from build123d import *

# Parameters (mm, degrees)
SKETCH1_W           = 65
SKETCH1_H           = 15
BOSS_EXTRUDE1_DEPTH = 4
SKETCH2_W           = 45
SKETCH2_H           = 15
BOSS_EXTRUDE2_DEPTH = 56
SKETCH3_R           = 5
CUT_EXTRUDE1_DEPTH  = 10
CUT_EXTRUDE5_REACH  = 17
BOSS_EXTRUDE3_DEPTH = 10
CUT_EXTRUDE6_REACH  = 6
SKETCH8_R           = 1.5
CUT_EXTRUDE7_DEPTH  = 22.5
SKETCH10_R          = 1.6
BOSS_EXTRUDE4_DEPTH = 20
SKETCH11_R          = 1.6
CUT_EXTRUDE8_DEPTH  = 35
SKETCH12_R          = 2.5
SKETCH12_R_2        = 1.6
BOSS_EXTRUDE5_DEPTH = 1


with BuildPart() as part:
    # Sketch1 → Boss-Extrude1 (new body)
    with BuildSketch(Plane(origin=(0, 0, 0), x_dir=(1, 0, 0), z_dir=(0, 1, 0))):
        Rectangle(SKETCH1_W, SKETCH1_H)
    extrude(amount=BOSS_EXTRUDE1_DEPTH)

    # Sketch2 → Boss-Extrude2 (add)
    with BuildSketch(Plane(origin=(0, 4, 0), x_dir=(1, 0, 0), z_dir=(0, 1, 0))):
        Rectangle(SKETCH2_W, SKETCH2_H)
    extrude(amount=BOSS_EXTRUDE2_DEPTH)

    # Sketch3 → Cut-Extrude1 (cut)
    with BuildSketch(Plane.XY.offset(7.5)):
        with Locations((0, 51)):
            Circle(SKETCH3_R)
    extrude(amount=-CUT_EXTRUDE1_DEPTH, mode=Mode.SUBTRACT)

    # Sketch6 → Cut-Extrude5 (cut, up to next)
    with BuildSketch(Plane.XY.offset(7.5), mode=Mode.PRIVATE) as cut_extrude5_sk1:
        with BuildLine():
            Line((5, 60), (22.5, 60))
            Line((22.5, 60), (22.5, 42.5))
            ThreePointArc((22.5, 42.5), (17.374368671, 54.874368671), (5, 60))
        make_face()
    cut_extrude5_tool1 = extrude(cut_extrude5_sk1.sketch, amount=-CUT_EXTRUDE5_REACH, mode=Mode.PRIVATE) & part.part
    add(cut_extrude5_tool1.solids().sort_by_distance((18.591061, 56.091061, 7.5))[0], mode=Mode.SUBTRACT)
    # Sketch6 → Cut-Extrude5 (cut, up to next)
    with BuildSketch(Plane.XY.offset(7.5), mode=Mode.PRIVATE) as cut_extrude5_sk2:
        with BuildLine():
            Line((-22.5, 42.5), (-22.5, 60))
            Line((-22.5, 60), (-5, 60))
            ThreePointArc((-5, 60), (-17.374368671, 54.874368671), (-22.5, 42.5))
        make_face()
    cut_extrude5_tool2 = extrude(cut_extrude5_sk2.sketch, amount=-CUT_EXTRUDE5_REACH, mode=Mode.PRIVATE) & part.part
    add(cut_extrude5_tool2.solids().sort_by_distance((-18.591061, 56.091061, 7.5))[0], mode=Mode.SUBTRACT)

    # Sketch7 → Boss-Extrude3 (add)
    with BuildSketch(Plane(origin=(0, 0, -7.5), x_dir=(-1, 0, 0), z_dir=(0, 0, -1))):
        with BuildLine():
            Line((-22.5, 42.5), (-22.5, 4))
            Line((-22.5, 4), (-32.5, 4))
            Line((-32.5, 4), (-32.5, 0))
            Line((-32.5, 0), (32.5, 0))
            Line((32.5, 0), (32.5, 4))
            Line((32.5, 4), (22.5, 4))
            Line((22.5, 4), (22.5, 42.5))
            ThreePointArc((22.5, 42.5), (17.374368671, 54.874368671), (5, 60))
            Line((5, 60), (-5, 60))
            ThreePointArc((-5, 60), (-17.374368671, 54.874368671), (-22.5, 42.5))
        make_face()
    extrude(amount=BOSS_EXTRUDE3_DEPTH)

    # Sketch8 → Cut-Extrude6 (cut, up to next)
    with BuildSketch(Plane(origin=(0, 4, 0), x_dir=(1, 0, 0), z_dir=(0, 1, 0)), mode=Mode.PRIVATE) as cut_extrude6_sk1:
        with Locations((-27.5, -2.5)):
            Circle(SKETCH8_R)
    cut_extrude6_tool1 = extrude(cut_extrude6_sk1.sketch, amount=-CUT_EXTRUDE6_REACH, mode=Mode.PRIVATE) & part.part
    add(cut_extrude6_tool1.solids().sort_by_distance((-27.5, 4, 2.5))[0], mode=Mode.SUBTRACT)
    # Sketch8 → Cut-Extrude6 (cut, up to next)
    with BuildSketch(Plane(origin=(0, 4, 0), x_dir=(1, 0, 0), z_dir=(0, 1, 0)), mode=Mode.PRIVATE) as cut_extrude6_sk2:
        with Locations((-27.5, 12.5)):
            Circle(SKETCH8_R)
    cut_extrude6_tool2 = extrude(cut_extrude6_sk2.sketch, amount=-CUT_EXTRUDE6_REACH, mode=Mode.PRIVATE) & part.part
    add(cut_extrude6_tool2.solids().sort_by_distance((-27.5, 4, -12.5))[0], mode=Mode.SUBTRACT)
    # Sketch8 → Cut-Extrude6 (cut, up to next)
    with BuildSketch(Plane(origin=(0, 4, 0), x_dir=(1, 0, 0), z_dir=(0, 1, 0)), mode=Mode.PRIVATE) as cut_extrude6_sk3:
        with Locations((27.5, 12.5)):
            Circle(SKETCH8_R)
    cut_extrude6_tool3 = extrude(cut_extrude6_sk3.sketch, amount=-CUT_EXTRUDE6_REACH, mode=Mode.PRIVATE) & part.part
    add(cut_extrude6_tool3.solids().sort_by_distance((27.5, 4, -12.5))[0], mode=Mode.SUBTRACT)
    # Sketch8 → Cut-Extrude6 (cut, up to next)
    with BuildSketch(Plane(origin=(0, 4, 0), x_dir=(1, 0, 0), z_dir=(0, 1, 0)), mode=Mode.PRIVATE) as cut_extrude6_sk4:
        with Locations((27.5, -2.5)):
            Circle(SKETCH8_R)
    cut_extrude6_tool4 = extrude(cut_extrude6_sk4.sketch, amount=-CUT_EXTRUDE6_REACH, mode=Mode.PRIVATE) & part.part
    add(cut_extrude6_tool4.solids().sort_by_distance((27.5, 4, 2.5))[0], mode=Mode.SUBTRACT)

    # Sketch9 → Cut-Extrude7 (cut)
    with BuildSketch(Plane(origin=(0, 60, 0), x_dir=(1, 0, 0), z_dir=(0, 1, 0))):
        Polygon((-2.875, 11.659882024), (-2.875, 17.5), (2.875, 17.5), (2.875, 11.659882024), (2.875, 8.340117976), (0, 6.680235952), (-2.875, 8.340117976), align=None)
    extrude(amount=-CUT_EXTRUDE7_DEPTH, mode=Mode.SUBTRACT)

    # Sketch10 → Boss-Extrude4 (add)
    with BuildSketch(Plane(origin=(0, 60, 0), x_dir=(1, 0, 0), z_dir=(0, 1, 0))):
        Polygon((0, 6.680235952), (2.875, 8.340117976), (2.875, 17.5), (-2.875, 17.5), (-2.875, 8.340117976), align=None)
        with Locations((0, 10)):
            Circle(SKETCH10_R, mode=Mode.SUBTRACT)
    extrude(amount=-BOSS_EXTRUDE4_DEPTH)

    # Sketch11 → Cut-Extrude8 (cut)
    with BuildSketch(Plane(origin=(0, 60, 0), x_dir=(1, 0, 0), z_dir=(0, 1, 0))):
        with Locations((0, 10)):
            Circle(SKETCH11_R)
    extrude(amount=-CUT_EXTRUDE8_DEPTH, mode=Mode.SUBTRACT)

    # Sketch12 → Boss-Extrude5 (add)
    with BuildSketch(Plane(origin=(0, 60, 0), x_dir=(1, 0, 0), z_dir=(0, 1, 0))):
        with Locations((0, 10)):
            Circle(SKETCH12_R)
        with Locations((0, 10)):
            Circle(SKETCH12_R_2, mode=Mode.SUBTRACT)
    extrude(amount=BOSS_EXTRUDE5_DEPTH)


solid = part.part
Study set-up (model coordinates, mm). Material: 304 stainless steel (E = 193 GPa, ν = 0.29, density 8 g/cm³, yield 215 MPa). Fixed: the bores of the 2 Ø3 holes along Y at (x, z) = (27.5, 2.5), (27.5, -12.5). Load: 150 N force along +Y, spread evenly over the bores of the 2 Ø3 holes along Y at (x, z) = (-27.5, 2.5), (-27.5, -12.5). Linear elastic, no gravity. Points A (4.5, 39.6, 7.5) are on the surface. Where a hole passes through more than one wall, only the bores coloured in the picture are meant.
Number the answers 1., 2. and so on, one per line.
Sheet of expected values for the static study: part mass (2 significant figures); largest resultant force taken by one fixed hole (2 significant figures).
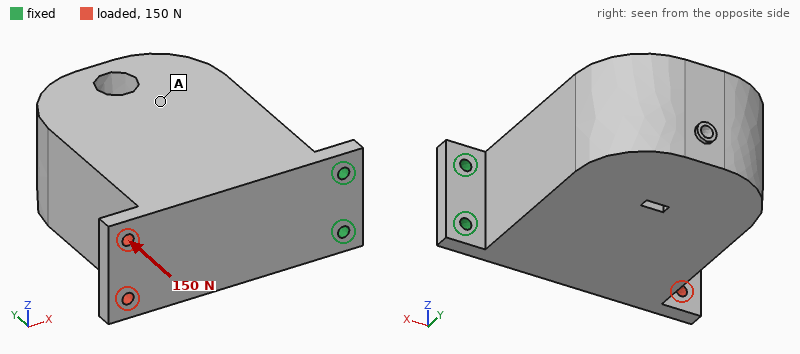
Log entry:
1. 520 g
2. 75 N
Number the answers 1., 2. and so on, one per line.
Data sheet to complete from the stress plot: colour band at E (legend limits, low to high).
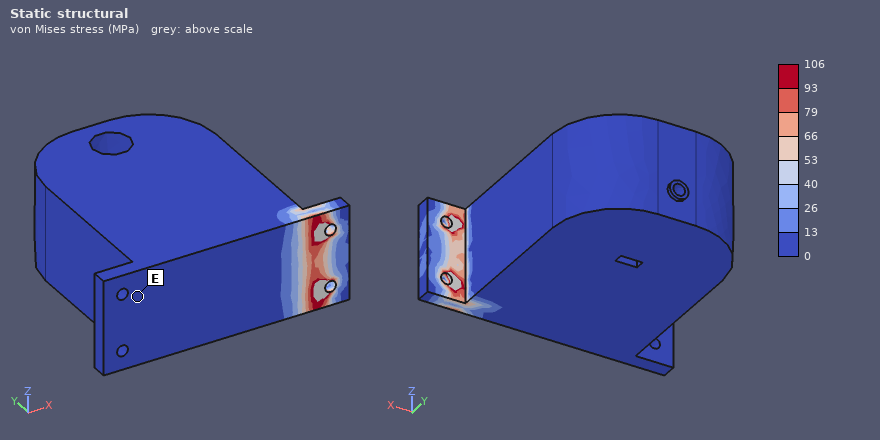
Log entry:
1. 0 to 13 MPa
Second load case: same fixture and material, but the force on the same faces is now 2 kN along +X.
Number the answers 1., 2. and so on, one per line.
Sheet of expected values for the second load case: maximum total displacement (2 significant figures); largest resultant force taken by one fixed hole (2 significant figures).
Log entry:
1. 12 µm
2. 1.0 kN
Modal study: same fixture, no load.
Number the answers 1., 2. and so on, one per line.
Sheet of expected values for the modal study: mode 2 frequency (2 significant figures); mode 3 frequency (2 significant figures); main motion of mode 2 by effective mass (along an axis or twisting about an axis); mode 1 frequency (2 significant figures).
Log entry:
1. 1100 Hz
2. 2800 Hz
3. along Z
4. 320 Hz
